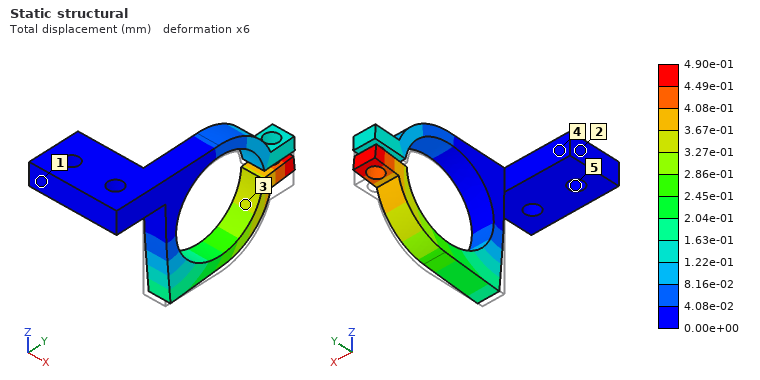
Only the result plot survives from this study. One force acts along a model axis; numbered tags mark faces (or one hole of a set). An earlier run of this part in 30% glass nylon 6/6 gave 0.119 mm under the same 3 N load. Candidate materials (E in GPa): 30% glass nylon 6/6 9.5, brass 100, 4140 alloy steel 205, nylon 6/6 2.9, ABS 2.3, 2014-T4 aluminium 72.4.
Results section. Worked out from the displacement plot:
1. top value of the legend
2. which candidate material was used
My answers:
4.90e-01 mm
ABS
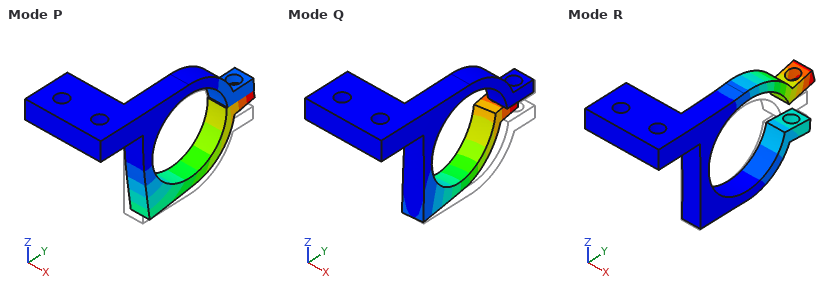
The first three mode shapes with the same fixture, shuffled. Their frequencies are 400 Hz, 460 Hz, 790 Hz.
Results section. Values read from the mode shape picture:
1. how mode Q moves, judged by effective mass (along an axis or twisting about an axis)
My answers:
along X
